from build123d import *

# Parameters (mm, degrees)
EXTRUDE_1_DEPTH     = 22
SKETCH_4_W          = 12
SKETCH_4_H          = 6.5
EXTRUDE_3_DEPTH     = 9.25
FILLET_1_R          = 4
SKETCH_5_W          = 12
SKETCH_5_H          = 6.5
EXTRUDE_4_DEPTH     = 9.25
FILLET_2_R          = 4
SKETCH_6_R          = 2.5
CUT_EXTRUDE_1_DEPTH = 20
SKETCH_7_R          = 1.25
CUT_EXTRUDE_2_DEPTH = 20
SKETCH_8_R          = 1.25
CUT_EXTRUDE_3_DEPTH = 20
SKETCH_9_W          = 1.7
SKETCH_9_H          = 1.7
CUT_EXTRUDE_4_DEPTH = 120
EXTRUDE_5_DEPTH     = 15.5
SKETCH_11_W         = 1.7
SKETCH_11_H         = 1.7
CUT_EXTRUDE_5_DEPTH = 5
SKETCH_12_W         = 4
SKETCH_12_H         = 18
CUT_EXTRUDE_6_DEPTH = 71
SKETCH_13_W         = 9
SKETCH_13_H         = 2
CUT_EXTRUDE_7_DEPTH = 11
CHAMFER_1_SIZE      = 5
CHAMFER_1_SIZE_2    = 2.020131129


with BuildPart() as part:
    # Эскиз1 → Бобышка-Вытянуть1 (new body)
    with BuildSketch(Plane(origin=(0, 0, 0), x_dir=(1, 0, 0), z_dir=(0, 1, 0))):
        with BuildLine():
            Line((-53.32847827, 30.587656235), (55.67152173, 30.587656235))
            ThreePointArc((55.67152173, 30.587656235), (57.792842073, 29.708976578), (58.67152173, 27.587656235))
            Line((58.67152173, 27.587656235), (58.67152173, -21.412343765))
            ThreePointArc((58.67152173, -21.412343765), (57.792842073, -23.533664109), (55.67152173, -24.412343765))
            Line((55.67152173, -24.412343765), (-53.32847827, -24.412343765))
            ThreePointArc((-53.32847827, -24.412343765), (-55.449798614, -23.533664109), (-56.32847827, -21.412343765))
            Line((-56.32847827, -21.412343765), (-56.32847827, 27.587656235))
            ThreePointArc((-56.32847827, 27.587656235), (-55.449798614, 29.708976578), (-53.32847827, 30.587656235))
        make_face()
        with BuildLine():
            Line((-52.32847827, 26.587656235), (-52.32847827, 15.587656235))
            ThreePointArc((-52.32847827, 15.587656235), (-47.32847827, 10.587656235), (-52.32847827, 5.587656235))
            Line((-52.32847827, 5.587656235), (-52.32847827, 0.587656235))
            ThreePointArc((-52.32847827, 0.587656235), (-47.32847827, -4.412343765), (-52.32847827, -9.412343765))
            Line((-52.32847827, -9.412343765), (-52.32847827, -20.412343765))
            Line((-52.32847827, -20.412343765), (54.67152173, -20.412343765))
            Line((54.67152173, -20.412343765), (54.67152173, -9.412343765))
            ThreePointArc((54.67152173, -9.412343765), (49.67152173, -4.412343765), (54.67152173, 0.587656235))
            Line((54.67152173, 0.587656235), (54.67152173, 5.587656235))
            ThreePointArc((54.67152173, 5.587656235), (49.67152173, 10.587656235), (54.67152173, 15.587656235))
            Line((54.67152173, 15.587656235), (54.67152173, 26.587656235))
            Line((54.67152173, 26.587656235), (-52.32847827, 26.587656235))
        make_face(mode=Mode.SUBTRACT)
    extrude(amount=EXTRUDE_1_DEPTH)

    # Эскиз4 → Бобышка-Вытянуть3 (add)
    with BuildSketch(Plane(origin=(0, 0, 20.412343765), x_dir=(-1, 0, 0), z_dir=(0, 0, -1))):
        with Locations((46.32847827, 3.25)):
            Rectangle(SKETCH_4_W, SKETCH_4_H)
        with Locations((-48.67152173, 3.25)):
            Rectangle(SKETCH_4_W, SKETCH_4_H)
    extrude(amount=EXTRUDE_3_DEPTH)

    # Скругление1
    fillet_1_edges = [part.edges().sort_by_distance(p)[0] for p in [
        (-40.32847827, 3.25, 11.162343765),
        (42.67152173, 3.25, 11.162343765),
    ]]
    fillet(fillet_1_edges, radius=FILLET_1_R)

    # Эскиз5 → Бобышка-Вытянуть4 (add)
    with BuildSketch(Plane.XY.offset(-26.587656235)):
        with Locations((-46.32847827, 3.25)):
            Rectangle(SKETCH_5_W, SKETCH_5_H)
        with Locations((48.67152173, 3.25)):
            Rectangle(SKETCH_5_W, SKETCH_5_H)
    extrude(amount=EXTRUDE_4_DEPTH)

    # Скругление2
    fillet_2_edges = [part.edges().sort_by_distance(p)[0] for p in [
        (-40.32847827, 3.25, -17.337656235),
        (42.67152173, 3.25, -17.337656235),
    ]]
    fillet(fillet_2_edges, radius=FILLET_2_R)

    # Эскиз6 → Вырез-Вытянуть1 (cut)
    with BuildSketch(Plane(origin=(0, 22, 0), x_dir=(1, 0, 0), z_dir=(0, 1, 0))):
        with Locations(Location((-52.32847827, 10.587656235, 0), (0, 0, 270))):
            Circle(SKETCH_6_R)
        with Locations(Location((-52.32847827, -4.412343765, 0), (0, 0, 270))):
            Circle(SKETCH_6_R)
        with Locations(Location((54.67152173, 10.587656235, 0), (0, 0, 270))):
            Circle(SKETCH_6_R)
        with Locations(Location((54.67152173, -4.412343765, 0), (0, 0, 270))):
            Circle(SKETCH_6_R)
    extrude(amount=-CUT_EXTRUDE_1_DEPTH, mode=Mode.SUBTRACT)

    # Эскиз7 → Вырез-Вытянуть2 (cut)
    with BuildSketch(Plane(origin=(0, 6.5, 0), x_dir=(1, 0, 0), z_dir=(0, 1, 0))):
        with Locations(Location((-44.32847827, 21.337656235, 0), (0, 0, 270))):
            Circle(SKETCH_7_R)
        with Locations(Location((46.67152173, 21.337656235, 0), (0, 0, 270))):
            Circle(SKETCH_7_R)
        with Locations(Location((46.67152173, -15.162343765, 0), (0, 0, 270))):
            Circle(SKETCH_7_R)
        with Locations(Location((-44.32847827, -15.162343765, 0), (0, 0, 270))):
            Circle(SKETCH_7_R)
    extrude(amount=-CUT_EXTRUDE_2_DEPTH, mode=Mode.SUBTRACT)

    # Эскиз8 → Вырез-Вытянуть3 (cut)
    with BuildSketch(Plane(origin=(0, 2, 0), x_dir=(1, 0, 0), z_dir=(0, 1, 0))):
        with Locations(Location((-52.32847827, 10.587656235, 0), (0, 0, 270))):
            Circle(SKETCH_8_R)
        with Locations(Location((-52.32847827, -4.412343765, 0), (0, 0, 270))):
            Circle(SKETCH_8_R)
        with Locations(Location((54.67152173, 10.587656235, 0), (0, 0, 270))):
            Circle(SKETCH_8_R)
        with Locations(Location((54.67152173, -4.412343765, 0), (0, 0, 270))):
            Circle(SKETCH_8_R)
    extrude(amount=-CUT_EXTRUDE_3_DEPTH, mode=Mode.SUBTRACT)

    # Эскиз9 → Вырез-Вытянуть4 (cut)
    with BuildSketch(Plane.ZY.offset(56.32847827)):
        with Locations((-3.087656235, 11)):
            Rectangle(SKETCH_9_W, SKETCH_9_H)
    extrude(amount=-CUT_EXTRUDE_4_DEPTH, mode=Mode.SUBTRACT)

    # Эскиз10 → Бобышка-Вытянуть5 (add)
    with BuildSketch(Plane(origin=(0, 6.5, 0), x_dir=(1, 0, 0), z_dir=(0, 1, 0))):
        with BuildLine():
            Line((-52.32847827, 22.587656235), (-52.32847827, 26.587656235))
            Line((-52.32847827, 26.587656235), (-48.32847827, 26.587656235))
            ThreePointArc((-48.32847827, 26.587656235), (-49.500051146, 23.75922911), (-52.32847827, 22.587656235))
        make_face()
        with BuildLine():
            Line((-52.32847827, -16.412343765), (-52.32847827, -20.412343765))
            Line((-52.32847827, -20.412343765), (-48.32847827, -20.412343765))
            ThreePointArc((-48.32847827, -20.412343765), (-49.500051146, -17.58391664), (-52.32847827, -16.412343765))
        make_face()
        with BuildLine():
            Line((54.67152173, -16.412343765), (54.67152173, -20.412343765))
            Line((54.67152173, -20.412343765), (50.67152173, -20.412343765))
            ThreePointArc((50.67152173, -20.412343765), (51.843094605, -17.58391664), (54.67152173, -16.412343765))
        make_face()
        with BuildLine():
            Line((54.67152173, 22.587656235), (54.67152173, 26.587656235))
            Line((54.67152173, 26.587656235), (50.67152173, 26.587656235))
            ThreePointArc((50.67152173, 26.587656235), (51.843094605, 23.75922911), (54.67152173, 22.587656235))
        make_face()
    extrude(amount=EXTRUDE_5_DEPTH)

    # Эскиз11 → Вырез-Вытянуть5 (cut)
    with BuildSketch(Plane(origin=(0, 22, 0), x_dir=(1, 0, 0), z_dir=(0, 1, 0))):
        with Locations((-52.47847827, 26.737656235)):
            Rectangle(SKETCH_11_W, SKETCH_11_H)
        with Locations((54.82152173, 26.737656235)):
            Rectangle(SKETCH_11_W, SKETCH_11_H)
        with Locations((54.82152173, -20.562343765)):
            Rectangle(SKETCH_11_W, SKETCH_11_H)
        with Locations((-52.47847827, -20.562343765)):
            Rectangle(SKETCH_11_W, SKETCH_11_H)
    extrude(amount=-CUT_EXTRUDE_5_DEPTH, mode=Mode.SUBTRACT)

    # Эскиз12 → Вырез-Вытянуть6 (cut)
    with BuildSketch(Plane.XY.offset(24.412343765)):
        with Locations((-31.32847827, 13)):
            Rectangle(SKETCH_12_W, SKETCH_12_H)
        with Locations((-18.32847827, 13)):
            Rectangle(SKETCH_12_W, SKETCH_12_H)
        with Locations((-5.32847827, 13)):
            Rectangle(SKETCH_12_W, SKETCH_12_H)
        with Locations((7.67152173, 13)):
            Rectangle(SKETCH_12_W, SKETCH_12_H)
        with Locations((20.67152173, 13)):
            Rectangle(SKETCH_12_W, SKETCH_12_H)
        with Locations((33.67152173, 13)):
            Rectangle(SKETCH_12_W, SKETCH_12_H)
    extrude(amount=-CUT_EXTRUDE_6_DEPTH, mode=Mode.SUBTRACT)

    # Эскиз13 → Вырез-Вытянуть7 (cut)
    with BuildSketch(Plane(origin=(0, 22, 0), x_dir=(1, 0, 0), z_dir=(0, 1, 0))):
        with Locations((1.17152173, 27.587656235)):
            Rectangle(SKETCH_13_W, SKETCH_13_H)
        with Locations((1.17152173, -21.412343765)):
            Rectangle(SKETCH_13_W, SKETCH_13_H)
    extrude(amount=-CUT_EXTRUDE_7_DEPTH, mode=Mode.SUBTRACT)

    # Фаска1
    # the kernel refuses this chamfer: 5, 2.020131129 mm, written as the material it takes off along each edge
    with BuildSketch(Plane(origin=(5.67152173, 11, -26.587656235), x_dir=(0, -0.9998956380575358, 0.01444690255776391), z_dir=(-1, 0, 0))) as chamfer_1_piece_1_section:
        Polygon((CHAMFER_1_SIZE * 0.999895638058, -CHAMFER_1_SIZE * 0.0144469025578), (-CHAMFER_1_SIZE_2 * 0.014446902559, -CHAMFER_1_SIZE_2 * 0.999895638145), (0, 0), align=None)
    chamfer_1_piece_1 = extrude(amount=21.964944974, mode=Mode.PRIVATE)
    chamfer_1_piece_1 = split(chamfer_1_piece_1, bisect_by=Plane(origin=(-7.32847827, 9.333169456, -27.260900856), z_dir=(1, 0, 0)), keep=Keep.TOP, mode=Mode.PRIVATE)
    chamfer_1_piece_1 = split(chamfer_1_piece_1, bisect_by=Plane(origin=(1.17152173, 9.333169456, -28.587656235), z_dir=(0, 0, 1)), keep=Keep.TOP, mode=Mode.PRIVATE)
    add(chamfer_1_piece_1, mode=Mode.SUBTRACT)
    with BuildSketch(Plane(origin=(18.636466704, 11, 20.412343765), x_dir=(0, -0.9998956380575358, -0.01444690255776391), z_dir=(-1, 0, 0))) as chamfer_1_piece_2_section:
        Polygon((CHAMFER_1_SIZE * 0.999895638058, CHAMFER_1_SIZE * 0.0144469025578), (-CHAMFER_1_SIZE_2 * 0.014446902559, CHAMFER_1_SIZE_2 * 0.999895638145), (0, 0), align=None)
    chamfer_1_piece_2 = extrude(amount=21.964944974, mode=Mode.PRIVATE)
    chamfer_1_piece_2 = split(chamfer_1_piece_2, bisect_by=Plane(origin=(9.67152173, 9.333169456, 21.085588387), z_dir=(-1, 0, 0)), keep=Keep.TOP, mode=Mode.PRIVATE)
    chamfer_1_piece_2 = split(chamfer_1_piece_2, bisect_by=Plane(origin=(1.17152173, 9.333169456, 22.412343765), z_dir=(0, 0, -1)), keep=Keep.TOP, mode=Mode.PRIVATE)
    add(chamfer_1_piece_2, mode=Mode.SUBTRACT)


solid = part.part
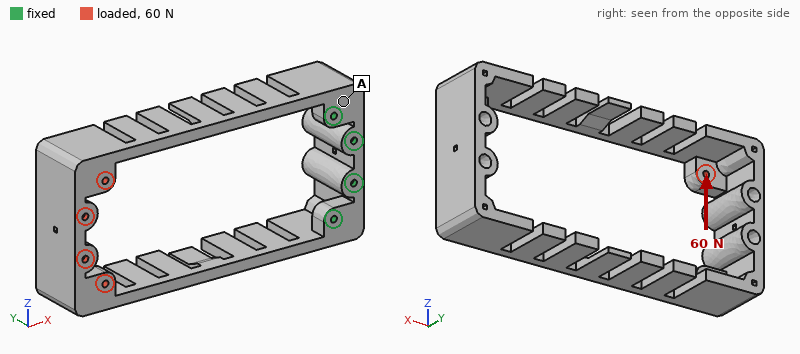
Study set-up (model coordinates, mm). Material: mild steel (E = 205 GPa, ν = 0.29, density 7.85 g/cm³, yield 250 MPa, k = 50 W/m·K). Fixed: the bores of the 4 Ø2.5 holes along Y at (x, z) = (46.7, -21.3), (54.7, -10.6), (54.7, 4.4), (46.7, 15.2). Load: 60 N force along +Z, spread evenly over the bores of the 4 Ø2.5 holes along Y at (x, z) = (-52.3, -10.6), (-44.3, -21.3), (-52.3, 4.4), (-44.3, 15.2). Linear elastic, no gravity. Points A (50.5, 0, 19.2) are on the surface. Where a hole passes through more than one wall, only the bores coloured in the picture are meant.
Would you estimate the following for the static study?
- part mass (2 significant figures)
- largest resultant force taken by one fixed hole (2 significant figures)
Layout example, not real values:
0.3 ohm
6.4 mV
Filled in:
230 g
170 N
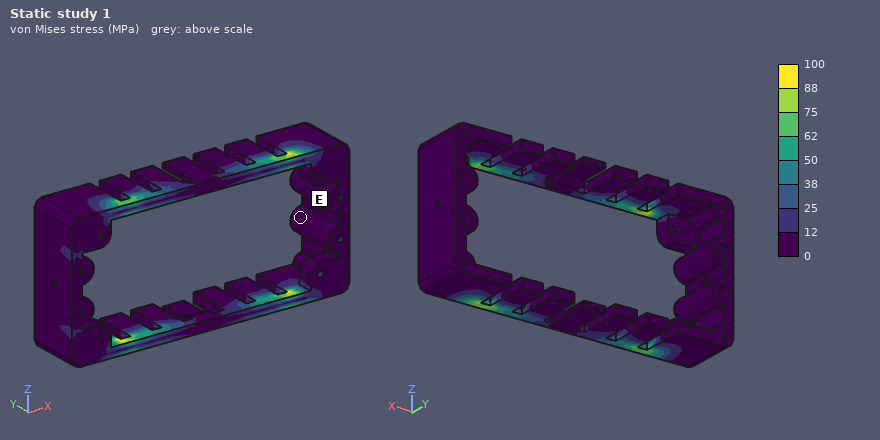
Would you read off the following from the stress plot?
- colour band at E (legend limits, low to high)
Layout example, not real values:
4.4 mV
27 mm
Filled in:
0 to 12 MPa
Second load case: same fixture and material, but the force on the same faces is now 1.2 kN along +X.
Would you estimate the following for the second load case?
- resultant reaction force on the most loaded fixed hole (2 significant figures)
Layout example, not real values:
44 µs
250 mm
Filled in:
730 N
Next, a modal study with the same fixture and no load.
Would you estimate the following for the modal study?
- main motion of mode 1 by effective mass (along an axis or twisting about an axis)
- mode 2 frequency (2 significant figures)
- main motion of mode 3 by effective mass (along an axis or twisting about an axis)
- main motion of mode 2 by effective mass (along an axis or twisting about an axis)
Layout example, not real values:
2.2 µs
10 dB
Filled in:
along Y
220 Hz
twisting about X
along Z
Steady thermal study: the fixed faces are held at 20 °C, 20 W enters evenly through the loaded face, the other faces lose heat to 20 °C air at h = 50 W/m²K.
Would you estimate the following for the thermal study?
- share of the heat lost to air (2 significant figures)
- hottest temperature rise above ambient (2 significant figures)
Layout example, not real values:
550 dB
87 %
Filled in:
99 %
68 K
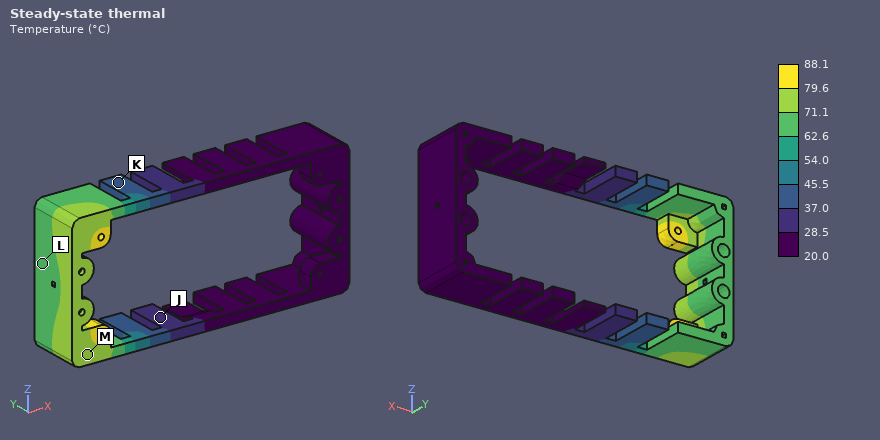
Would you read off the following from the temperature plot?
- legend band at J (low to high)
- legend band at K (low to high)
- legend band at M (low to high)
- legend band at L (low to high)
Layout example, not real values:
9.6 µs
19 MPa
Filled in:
28.5 to 37.0 °C
37.0 to 45.5 °C
71.1 to 79.6 °C
62.6 to 71.1 °C
